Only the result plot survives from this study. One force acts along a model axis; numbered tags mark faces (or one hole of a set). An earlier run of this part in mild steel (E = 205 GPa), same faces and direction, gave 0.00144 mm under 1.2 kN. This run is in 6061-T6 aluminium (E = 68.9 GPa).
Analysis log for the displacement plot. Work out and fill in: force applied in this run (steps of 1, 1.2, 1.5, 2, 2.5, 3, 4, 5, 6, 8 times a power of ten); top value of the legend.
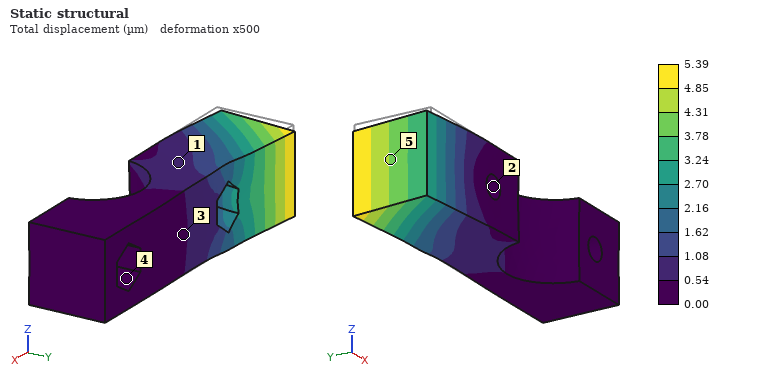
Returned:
1.5 kN
5.39 µm
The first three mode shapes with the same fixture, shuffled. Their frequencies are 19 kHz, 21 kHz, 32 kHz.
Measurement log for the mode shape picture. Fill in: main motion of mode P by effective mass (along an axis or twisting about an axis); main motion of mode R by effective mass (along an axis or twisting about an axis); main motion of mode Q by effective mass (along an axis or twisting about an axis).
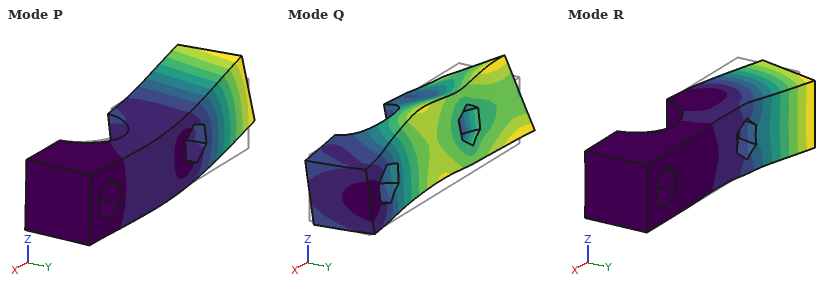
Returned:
along Z
along Y
along Z
